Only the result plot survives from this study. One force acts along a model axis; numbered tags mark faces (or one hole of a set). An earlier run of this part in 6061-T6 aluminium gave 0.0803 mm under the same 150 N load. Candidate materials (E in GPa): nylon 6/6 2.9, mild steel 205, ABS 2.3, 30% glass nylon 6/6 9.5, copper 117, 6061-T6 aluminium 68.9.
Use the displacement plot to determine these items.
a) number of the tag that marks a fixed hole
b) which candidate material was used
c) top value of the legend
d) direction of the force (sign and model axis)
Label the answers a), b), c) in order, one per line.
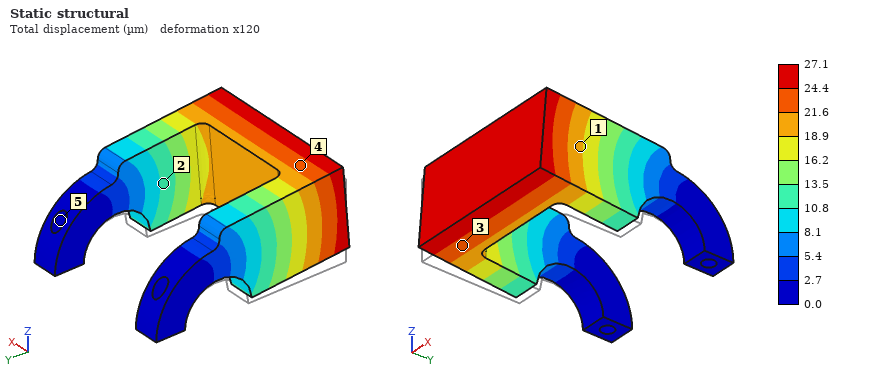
a) 5
b) mild steel
c) 27.1 µm
d) +Z
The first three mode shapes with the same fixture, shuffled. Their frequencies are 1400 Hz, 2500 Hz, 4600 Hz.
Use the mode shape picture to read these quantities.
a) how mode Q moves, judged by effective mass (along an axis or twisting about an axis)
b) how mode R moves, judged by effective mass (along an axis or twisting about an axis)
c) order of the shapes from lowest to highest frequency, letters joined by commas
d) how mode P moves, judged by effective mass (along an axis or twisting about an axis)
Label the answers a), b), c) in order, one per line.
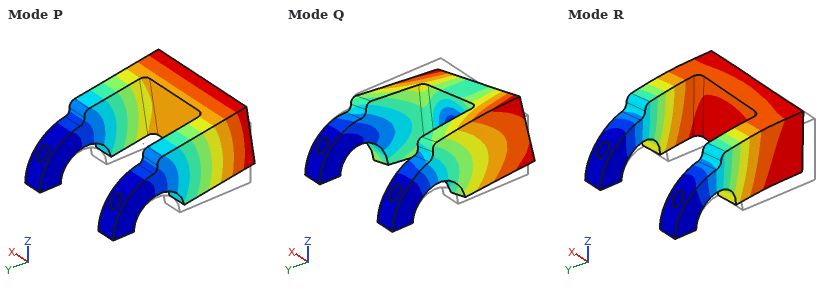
a) twisting about Y
b) along X
c) P, R, Q
d) along Z
